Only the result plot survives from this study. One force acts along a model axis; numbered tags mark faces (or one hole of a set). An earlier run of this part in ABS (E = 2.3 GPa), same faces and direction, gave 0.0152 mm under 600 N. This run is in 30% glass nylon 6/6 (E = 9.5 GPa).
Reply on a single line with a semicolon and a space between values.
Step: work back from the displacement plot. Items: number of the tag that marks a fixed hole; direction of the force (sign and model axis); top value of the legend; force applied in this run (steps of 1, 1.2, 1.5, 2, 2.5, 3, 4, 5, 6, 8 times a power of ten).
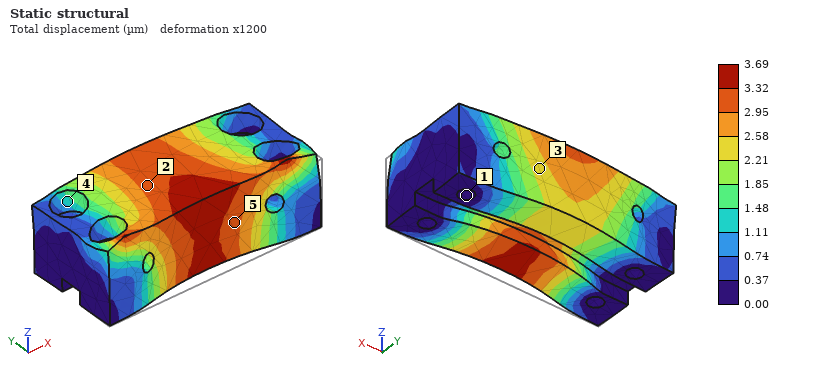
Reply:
1; +Y; 3.69 µm; 600 N
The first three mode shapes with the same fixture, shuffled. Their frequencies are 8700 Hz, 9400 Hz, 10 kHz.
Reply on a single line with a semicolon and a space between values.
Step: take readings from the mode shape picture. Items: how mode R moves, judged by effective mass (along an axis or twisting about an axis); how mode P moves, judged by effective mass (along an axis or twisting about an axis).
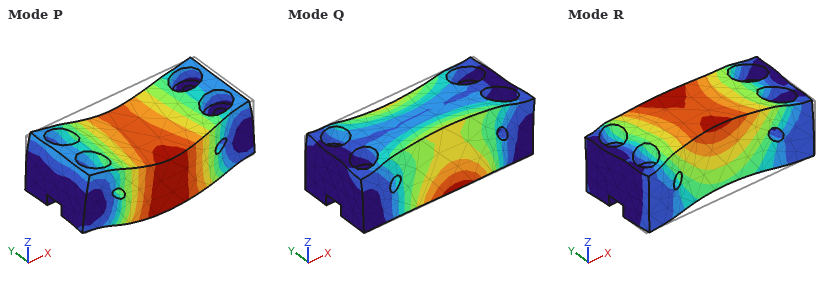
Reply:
along Y; along Z
